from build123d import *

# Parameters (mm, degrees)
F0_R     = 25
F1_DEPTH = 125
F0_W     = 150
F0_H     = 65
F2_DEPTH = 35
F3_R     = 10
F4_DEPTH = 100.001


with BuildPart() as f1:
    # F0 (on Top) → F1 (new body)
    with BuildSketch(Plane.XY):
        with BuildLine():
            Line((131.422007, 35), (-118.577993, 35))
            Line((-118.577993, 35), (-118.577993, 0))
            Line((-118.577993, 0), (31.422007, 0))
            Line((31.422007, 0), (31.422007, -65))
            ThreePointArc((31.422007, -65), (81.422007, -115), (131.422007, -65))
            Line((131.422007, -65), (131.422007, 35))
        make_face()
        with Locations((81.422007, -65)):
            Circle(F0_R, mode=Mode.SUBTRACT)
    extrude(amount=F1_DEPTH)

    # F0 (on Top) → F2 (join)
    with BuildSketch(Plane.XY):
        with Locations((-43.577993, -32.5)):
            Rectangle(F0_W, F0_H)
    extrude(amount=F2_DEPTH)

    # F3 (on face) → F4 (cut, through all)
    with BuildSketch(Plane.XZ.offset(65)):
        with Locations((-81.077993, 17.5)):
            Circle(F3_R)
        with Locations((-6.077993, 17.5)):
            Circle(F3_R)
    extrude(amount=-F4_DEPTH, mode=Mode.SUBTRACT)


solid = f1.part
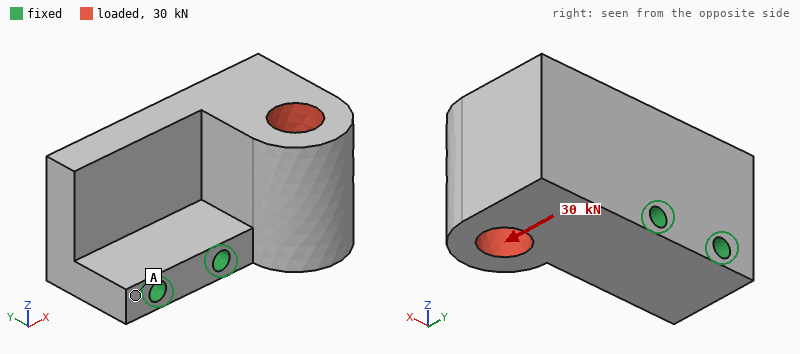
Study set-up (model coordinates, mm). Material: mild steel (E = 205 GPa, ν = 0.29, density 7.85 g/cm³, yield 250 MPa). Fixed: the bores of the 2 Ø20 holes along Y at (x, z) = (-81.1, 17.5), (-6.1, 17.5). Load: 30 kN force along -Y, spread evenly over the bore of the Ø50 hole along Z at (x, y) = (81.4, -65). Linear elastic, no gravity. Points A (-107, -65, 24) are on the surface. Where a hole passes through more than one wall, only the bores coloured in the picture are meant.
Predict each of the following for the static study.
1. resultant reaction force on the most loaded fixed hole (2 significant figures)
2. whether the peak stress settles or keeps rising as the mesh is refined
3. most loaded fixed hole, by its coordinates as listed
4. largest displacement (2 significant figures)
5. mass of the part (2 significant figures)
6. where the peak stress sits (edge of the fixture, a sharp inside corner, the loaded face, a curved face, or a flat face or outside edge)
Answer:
31 kN
keeps rising
(-6.1, 17.5)
45 µm
19 kg
edge of the fixture
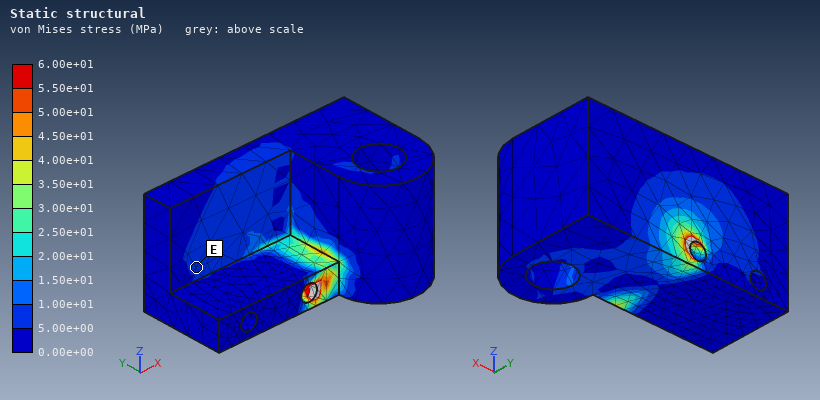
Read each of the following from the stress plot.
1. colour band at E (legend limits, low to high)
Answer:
5.00e+00 to 1.00e+01 MPa
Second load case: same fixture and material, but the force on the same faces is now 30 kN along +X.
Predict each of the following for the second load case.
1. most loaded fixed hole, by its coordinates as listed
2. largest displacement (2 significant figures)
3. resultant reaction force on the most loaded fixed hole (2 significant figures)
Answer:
(-6.1, 17.5)
48 µm
26 kN
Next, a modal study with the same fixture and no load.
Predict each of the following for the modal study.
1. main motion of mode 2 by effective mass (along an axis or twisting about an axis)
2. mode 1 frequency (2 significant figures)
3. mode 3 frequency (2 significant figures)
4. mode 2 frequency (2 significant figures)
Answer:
along Y
1300 Hz
2300 Hz
1400 Hz
